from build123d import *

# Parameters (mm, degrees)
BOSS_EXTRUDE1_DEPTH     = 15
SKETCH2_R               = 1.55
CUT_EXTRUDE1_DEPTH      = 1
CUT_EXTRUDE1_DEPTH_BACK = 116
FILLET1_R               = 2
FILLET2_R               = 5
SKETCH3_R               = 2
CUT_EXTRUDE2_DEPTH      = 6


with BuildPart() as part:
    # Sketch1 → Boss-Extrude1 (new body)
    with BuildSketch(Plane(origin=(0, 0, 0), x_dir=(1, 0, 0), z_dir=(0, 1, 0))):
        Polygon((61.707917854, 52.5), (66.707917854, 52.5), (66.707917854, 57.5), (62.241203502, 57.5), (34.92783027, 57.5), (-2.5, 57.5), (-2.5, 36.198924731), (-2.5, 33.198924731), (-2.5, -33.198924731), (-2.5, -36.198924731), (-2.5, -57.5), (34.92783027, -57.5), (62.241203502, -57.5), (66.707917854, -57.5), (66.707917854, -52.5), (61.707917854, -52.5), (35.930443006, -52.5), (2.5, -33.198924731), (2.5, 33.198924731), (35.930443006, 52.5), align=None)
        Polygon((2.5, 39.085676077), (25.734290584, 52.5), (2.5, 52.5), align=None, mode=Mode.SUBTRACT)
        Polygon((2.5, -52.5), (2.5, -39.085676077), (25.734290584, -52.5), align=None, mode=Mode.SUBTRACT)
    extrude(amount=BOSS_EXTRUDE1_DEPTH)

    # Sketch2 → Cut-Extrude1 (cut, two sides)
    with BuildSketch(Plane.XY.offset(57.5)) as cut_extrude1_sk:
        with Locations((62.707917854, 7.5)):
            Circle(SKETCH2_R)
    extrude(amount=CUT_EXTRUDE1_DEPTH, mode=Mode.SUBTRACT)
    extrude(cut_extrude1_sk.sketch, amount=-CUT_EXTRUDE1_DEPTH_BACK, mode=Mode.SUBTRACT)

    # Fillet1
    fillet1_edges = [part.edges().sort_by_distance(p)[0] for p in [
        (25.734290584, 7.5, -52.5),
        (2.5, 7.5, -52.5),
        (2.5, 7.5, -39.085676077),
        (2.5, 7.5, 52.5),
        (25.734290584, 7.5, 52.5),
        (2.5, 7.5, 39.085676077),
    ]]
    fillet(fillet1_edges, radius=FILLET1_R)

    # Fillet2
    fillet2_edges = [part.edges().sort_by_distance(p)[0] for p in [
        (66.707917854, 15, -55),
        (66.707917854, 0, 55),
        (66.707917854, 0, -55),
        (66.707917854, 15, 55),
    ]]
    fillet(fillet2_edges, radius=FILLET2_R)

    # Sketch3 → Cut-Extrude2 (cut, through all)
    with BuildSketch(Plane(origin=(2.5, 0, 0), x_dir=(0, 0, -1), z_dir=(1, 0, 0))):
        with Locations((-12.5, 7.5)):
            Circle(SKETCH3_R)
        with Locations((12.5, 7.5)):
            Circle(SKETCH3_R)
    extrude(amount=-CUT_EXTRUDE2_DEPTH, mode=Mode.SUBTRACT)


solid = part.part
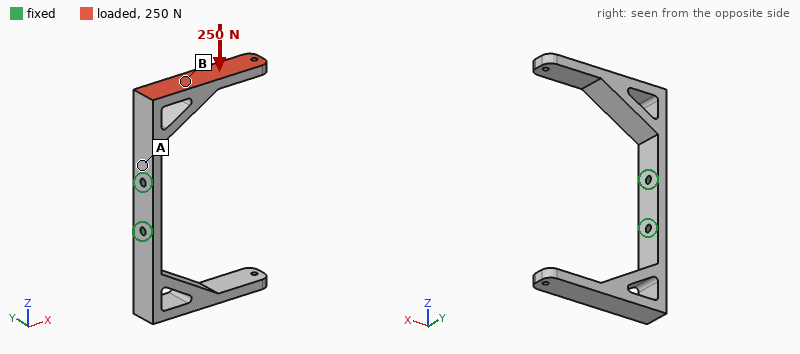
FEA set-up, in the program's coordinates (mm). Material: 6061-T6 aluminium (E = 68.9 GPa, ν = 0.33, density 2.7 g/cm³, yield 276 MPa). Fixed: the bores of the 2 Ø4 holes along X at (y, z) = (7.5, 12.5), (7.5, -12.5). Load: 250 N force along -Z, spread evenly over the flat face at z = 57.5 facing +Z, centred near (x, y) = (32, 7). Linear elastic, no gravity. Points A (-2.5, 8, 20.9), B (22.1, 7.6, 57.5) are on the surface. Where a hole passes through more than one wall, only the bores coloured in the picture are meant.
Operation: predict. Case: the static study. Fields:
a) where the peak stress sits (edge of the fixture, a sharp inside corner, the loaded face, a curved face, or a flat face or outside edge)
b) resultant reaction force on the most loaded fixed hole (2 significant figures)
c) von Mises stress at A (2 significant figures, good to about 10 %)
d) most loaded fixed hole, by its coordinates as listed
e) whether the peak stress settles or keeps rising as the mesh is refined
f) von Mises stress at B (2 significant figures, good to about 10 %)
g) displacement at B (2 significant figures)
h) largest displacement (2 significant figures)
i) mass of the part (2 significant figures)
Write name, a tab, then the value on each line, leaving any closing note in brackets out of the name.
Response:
where the peak stress sits	edge of the fixture
resultant reaction force on the most loaded fixed hole	230 N
von Mises stress at A	120 MPa
most loaded fixed hole, by its coordinates as listed	(7.5, 12.5)
whether the peak stress settles or keeps rising as the mesh is refined	keeps rising
von Mises stress at B	17 MPa
displacement at B	0.69 mm
largest displacement	1.4 mm
mass of the part	63 g
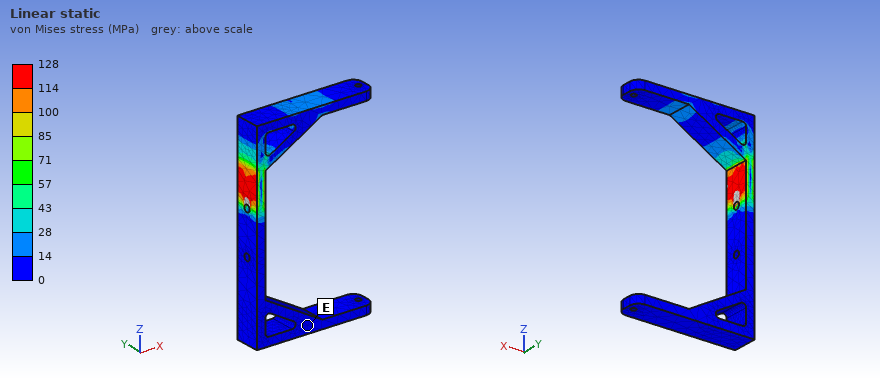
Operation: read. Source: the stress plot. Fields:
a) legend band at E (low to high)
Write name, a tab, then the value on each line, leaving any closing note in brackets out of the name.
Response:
legend band at E	0 to 14 MPa
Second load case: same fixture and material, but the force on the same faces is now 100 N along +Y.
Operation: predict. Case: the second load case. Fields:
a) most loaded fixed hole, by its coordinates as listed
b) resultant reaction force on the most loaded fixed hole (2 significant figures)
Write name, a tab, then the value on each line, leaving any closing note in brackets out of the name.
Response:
most loaded fixed hole, by its coordinates as listed	(7.5, 12.5)
resultant reaction force on the most loaded fixed hole	210 N
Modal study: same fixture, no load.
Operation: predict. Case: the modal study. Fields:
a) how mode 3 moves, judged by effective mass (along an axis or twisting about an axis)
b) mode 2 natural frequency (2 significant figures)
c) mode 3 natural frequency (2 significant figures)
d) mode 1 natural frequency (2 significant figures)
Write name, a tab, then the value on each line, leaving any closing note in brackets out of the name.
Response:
how mode 3 moves, judged by effective mass	along Y
mode 2 natural frequency	540 Hz
mode 3 natural frequency	790 Hz
mode 1 natural frequency	540 Hz
